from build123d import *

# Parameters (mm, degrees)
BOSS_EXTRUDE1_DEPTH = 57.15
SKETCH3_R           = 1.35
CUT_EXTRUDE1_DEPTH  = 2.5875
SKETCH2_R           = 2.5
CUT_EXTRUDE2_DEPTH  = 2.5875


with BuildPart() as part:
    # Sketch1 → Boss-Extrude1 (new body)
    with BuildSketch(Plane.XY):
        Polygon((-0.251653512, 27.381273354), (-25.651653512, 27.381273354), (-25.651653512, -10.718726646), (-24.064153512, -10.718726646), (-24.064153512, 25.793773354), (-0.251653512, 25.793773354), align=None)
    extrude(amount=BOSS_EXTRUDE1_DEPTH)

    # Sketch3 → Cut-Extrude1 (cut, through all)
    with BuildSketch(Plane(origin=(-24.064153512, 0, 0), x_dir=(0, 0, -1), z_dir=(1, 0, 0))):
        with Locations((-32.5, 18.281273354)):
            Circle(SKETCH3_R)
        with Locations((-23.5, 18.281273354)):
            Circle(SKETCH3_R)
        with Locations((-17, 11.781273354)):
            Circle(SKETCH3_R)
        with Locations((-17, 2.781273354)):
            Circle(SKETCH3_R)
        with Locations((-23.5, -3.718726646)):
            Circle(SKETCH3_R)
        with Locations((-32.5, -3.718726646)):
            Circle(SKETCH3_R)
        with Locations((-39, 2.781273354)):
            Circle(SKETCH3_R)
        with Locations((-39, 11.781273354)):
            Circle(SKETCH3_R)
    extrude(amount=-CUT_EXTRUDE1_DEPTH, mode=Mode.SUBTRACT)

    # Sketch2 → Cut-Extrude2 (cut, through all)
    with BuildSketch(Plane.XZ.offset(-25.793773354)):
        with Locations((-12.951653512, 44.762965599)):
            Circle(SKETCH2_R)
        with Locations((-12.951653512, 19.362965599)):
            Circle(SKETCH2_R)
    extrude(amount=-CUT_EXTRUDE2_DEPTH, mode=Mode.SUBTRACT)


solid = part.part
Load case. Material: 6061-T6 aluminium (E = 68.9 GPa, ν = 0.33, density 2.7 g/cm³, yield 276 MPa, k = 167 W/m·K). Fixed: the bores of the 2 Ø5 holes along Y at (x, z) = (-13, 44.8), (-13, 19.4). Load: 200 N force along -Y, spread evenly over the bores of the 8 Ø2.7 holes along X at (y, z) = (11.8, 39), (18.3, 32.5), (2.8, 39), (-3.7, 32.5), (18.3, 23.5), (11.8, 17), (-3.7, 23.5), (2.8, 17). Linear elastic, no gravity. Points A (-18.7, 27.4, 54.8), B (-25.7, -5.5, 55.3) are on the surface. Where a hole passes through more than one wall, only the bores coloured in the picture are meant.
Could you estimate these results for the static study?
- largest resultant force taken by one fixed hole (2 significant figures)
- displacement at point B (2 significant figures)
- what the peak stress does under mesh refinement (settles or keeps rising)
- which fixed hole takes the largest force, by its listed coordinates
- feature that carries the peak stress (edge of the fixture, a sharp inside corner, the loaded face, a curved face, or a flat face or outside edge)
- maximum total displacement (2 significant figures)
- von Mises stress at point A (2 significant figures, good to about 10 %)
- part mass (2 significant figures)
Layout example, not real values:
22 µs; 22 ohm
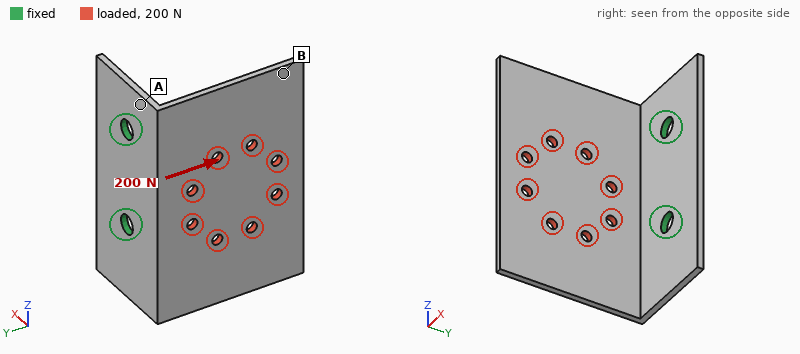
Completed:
130 N; 0.30 mm; keeps rising; (-13, 19.4); edge of the fixture; 0.39 mm; 35 MPa; 15 g
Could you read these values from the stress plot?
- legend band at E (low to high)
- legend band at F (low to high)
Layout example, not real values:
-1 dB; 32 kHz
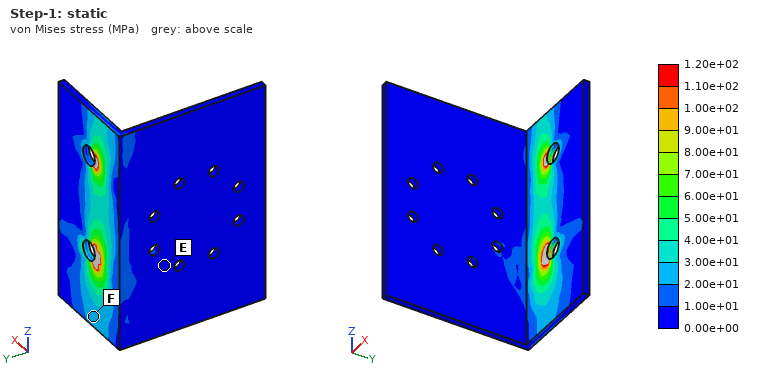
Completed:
0.00e+00 to 1.00e+01 MPa; 2.00e+01 to 3.00e+01 MPa
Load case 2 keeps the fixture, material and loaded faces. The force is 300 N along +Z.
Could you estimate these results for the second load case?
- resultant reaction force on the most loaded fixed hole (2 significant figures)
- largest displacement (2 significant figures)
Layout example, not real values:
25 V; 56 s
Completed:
270 N; 0.41 mm
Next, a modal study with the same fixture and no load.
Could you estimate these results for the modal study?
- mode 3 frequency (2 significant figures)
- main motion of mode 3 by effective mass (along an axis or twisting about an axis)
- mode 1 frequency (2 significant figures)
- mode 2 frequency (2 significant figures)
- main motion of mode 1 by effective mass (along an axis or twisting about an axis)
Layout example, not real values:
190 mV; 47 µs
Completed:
2100 Hz; along Z; 650 Hz; 1300 Hz; along X
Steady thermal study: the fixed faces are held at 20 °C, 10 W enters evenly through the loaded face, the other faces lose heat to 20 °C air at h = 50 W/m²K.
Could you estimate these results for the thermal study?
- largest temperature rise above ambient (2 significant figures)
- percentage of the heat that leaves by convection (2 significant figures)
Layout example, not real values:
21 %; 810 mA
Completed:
18 K; 32 %
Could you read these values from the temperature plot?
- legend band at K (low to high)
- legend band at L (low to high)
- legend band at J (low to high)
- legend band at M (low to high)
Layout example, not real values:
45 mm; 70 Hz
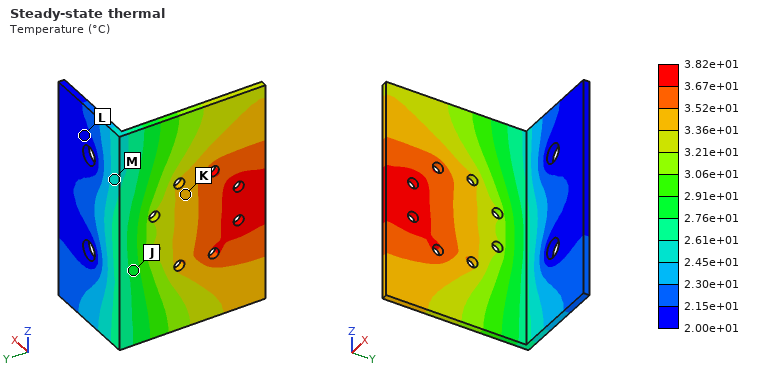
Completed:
3.36e+01 to 3.52e+01 °C; 2.00e+01 to 2.15e+01 °C; 2.76e+01 to 2.91e+01 °C; 2.45e+01 to 2.61e+01 °C
